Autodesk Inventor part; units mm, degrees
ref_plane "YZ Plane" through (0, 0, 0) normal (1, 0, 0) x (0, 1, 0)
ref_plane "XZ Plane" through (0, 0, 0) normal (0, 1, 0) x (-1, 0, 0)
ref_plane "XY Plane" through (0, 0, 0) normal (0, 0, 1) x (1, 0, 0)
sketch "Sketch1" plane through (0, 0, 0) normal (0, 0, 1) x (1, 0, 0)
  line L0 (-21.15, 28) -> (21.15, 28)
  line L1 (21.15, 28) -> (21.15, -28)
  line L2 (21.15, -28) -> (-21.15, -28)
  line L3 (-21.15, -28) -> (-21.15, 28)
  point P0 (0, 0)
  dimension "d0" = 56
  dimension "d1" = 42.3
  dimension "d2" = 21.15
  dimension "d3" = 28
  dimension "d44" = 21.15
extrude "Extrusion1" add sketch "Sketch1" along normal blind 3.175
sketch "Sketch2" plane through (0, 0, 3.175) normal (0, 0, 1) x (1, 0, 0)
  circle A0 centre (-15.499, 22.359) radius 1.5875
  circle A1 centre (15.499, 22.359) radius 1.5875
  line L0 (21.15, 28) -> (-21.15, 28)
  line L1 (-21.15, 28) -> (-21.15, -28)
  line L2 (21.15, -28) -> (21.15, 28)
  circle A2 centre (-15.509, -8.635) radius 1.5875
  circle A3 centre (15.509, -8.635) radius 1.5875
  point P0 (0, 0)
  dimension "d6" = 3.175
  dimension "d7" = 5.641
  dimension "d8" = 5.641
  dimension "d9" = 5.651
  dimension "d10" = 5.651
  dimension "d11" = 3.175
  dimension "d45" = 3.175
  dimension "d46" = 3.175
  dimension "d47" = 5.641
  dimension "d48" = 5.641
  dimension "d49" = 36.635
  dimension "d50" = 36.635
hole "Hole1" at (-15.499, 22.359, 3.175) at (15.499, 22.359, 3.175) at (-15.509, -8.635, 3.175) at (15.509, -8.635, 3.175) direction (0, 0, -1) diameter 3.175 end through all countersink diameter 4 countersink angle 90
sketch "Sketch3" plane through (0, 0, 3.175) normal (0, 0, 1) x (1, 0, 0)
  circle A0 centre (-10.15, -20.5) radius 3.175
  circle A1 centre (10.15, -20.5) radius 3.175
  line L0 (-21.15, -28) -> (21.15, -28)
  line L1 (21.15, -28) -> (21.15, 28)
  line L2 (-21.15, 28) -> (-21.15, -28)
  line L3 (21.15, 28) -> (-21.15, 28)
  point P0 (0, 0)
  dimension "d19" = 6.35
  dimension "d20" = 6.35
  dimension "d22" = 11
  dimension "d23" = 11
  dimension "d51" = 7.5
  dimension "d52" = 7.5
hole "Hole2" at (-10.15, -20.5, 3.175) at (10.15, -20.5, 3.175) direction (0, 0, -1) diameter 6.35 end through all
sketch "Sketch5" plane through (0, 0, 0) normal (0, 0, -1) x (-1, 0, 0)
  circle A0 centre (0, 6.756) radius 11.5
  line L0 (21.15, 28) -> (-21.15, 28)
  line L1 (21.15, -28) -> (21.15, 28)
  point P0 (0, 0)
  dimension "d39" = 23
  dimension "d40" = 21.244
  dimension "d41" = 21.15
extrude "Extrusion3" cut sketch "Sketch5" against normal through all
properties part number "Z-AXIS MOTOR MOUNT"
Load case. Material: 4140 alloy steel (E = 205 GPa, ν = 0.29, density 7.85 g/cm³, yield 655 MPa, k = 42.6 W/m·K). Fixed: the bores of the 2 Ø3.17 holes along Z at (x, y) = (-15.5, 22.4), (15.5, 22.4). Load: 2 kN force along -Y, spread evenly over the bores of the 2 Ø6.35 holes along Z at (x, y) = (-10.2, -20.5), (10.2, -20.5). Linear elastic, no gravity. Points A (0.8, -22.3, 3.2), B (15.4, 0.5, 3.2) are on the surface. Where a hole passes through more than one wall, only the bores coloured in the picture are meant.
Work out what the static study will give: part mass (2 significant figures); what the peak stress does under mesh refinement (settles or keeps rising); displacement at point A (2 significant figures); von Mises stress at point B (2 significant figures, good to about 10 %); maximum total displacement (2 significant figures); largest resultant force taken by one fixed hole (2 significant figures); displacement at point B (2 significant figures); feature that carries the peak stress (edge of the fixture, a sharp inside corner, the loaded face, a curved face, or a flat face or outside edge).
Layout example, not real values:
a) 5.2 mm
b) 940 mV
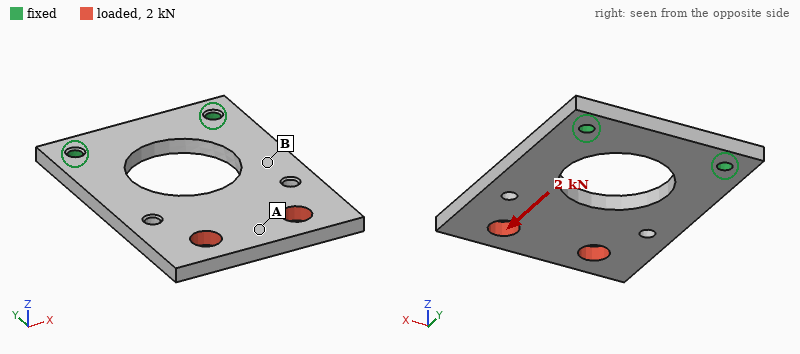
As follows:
a) 46 g
b) keeps rising
c) 7.0 µm
d) 27 MPa
e) 7.6 µm
f) 1.0 kN
g) 3.9 µm
h) edge of the fixture
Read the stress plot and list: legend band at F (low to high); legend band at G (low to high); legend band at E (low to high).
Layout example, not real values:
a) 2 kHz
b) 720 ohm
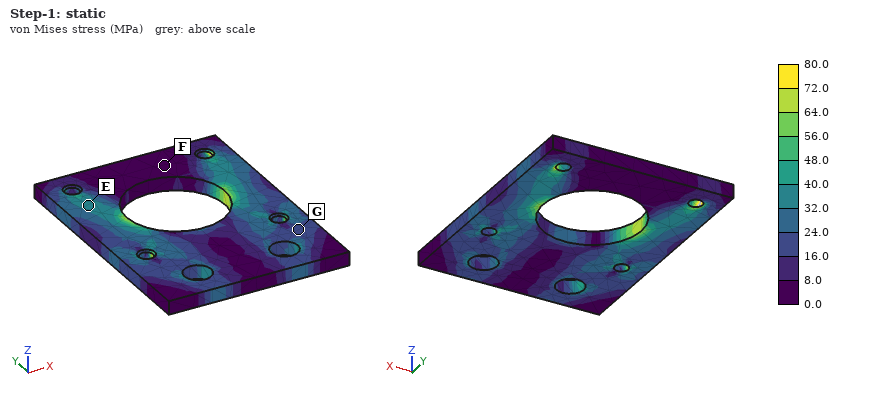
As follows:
a) 0.0 to 8.0 MPa
b) 16.0 to 24.0 MPa
c) 32.0 to 40.0 MPa
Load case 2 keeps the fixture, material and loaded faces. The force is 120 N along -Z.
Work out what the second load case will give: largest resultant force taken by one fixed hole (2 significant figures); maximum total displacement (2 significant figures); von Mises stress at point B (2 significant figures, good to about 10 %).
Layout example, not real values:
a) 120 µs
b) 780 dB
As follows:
a) 60 N
b) 0.31 mm
c) 68 MPa
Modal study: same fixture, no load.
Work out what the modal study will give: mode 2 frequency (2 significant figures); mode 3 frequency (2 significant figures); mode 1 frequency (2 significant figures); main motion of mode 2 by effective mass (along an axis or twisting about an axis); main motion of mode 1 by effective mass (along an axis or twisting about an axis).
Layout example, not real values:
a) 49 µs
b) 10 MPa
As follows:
a) 2500 Hz
b) 5800 Hz
c) 820 Hz
d) twisting about Y
e) along Z
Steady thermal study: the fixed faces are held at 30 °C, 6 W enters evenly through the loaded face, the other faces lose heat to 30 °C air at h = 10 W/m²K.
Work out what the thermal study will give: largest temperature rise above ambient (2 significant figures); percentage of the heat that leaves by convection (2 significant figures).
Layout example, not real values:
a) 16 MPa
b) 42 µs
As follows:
a) 63 K
b) 25 %
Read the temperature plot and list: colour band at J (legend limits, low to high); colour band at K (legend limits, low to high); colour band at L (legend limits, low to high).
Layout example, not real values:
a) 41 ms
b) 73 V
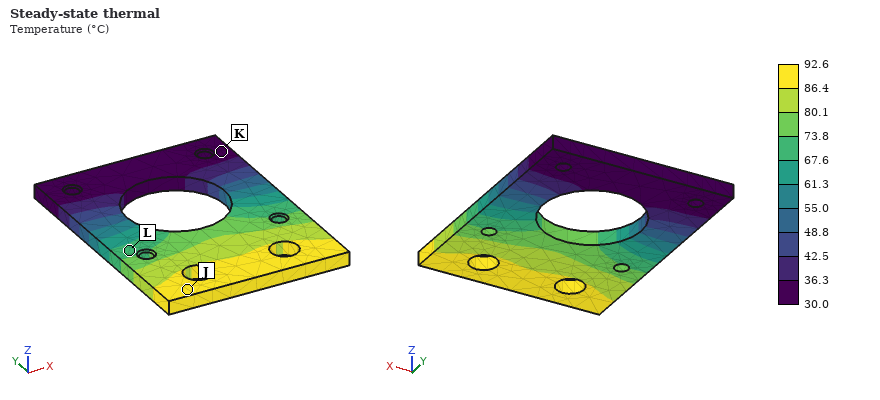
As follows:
a) 86.4 to 92.6 °C
b) 30.0 to 36.3 °C
c) 67.6 to 73.8 °C
